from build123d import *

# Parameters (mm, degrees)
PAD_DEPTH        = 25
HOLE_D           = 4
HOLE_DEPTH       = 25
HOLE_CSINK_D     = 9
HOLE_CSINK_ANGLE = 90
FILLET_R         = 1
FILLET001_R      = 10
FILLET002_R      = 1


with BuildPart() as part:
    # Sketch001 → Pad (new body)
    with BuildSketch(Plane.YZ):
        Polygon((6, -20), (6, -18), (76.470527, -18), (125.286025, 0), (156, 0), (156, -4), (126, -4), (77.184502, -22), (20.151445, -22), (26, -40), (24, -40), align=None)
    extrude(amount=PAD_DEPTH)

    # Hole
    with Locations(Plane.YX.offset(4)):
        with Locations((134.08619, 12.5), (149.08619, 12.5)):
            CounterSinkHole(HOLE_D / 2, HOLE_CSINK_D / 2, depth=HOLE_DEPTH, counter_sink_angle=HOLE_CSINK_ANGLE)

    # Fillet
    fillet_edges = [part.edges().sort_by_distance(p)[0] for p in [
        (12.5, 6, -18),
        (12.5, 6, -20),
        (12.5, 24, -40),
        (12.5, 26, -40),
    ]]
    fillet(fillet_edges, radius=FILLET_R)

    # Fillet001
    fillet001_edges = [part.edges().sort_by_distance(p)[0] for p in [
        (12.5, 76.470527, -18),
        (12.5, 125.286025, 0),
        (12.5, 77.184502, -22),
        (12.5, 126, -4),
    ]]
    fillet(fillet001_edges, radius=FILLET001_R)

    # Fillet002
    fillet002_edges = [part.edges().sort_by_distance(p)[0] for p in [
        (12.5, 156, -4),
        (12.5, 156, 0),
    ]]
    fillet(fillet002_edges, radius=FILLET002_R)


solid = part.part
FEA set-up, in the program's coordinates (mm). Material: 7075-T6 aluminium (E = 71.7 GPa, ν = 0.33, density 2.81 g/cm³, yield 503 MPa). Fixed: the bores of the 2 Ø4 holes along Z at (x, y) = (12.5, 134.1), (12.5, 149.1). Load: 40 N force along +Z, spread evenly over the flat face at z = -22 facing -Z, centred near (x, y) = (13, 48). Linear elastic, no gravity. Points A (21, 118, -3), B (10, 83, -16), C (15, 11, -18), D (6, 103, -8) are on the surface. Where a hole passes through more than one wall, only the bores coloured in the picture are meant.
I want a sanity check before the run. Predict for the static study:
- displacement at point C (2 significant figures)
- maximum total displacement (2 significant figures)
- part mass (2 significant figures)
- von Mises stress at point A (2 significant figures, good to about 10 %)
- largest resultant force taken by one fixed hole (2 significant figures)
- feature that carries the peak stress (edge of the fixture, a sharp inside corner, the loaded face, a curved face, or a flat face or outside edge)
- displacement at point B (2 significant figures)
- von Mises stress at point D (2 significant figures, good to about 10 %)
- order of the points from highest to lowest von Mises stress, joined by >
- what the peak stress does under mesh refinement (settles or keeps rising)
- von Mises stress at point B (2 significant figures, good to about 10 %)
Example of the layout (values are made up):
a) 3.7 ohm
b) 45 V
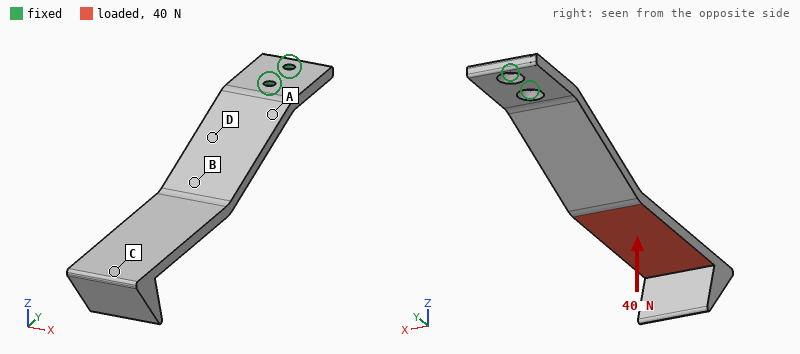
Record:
a) 1.7 mm
b) 1.8 mm
c) 51 g
d) 42 MPa
e) 330 N
f) edge of the fixture
g) 0.48 mm
h) 34 MPa
i) A > D > B > C
j) keeps rising
k) 22 MPa
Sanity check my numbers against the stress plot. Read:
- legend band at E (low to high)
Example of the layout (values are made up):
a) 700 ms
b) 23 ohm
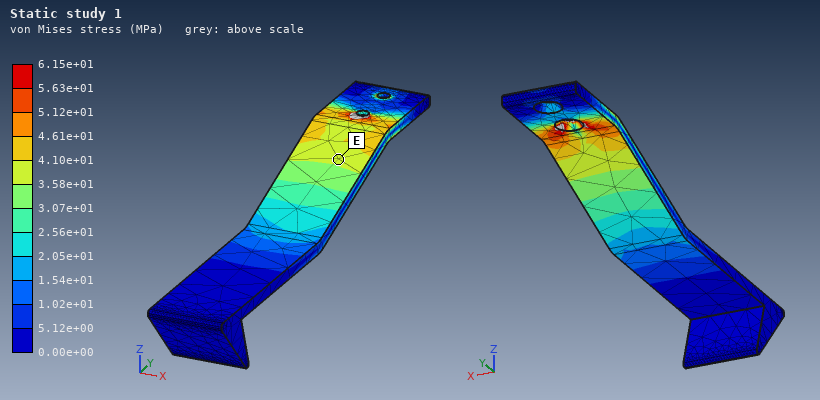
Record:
a) 3.58e+01 to 4.10e+01 MPa
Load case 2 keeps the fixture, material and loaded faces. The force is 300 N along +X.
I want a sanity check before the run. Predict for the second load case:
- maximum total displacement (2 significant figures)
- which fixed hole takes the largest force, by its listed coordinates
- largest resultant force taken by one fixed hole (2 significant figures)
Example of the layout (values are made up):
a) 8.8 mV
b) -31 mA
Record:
a) 0.80 mm
b) (12.5, 134.1)
c) 1.6 kN
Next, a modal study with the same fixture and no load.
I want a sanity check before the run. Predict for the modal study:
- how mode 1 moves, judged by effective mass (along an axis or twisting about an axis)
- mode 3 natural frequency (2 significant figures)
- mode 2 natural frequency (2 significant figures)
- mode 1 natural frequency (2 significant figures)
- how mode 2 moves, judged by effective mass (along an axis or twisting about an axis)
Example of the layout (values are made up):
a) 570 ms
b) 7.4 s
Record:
a) along Z
b) 980 Hz
c) 570 Hz
d) 140 Hz
e) along X
